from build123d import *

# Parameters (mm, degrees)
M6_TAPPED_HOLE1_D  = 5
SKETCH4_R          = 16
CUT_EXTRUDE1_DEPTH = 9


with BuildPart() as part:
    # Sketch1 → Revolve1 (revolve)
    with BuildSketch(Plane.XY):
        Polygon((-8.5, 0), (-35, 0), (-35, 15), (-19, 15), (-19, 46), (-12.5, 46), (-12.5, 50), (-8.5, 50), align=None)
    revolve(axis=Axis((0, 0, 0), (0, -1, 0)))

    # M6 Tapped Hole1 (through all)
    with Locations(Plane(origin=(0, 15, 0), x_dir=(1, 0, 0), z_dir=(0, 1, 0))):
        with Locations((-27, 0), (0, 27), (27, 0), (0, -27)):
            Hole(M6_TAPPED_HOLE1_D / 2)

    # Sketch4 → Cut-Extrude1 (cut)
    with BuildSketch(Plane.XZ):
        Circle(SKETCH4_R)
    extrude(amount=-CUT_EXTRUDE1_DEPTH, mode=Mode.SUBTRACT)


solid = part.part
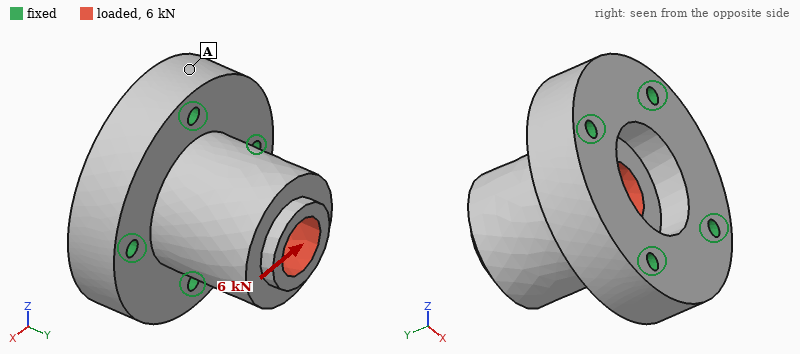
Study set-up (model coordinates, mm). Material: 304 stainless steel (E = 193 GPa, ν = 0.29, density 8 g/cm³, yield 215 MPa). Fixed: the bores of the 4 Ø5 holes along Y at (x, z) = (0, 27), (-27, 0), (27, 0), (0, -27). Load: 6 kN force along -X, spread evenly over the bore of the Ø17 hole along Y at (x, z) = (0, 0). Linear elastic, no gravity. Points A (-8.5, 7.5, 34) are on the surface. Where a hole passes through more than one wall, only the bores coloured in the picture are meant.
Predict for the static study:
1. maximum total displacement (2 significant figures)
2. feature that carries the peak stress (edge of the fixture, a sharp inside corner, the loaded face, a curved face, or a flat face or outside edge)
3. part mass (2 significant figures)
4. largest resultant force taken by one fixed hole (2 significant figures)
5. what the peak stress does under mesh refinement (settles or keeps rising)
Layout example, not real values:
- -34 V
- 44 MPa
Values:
- 7.7 µm
- edge of the fixture
- 620 g
- 3.0 kN
- keeps rising
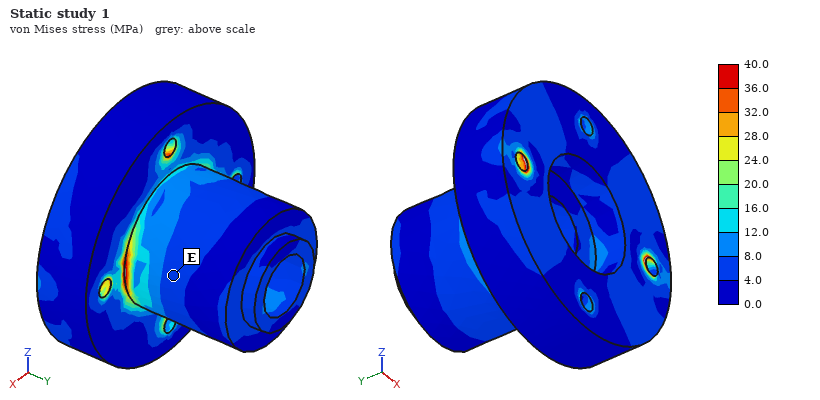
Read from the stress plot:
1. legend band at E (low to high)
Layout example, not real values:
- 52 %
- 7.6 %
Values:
- 4.0 to 8.0 MPa
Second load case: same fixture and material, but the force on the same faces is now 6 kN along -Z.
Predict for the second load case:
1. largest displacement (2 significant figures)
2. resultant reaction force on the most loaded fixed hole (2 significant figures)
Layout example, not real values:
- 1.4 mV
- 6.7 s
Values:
- 7.7 µm
- 3.0 kN
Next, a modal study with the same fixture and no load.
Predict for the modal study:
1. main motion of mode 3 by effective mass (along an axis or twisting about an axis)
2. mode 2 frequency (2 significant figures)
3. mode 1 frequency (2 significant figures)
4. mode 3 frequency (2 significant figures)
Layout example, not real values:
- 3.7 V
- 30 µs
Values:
- along Y
- 11 kHz
- 10 kHz
- 17 kHz
